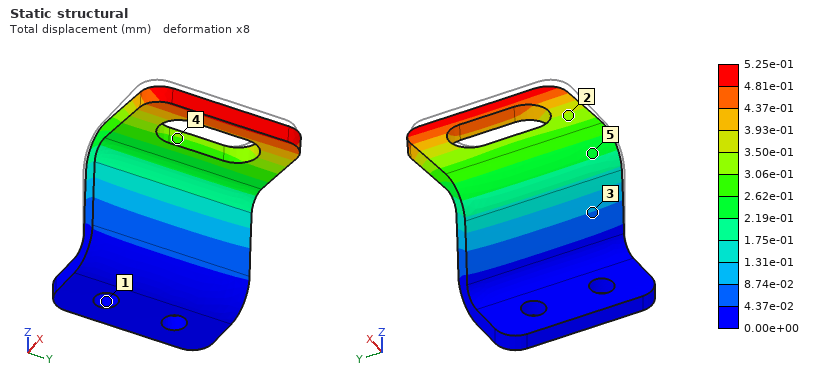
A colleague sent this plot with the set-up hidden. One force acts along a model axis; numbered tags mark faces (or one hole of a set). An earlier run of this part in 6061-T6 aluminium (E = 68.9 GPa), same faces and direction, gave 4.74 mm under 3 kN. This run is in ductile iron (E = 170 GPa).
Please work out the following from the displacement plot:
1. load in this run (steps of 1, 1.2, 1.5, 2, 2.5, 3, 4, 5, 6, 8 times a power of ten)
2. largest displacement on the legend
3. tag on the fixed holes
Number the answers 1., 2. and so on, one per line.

1. 800 N
2. 5.25e-01 mm
3. 1
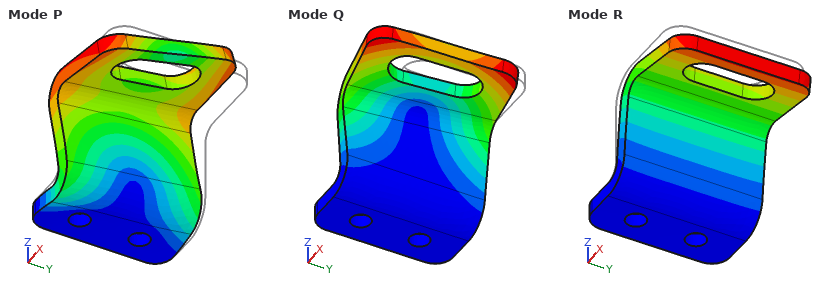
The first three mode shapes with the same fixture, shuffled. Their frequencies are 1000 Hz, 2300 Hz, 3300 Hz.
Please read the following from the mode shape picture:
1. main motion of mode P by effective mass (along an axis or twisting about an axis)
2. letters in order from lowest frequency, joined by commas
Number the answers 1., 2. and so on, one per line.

1. along Y
2. R, Q, P
